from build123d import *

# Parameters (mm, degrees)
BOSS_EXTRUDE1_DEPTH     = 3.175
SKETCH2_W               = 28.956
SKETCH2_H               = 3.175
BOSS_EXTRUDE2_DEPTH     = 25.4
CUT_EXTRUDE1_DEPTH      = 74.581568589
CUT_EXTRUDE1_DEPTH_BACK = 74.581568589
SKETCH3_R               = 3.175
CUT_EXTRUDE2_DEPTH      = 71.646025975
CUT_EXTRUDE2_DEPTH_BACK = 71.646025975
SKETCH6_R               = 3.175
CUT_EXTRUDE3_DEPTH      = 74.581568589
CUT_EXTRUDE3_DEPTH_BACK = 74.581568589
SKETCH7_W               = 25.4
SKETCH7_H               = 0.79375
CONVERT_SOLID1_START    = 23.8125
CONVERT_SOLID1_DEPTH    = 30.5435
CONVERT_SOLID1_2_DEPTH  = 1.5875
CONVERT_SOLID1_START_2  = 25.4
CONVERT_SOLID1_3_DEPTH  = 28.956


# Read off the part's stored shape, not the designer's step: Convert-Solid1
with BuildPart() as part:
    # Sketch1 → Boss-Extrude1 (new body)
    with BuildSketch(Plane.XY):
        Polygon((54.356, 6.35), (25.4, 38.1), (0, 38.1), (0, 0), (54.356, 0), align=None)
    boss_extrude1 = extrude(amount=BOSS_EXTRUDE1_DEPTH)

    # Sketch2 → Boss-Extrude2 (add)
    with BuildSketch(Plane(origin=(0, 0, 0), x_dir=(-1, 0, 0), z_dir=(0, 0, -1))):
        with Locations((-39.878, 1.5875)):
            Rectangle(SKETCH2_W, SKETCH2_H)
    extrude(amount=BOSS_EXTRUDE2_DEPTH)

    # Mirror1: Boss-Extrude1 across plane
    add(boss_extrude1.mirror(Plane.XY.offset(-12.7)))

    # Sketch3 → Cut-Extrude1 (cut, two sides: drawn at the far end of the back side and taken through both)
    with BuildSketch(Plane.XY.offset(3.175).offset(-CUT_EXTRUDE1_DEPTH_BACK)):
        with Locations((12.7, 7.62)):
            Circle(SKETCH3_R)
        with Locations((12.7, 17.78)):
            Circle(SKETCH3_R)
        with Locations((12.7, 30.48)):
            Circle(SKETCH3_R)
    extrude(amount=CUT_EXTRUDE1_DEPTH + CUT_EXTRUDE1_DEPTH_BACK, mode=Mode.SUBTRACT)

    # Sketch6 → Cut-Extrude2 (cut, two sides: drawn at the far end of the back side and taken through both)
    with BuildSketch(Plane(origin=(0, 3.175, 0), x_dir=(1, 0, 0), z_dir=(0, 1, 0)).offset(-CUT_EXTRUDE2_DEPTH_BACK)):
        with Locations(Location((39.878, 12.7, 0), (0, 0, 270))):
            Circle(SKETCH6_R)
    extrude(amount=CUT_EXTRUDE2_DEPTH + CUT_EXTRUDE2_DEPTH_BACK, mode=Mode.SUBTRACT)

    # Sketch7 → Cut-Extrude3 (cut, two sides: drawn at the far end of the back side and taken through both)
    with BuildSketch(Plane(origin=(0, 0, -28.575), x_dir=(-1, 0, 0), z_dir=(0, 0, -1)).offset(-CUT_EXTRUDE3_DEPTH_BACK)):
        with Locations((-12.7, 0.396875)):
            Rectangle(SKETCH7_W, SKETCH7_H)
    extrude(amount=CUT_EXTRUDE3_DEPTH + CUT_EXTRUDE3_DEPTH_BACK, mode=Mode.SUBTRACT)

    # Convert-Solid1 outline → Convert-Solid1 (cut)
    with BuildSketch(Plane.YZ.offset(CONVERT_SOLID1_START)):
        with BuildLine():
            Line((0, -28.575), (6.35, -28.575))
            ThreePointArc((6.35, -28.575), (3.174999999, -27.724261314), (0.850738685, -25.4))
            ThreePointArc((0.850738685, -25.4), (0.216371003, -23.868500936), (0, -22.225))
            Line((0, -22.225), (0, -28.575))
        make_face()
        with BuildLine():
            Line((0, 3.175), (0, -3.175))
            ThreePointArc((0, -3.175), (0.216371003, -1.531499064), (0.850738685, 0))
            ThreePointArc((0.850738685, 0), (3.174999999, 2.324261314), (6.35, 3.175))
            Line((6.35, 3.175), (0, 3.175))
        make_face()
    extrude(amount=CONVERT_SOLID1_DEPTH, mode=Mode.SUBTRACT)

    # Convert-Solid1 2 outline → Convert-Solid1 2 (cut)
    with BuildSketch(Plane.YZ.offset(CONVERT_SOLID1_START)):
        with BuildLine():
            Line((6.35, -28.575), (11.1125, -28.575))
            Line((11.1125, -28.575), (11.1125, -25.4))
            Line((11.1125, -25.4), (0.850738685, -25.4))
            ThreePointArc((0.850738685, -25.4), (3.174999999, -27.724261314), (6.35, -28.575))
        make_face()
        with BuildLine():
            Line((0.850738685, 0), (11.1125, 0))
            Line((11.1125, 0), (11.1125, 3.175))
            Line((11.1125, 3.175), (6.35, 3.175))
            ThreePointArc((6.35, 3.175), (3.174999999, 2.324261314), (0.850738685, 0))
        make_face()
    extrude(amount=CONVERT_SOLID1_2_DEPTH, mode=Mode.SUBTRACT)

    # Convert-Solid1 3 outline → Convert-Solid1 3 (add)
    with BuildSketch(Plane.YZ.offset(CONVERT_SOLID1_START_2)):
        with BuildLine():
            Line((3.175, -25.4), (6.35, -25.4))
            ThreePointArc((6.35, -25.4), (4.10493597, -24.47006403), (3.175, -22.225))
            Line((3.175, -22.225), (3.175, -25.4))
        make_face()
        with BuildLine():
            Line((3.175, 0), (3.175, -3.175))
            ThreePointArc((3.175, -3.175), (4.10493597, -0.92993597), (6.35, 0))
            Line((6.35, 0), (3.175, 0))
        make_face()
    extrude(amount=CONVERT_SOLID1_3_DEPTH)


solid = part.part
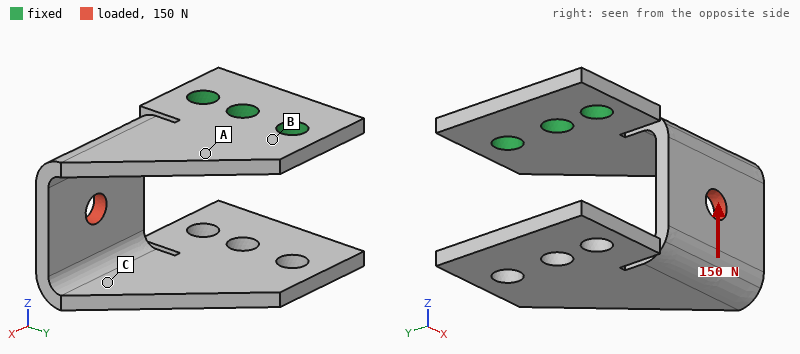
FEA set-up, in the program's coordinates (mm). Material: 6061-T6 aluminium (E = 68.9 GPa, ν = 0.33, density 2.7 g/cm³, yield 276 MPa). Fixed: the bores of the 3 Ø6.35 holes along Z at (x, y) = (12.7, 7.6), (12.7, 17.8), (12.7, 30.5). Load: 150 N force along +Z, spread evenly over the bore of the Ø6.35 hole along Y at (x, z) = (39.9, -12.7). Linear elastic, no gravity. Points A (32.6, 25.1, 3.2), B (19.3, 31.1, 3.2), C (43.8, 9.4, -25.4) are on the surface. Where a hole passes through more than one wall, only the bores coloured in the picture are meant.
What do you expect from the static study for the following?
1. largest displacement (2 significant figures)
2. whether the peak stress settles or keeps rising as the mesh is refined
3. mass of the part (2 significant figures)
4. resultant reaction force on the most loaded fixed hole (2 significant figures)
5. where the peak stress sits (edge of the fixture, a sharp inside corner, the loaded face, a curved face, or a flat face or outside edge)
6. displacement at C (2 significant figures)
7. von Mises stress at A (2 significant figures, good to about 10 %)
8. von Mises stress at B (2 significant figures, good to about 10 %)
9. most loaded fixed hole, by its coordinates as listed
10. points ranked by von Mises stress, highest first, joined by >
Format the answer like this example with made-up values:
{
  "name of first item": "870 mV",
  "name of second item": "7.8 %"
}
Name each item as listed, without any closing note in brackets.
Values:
{
  "largest displacement": "0.73 mm",
  "whether the peak stress settles or keeps rising as the mesh is refined": "keeps rising",
  "mass of the part": "30 g",
  "resultant reaction force on the most loaded fixed hole": "130 N",
  "where the peak stress sits": "a sharp inside corner",
  "displacement at C": "0.51 mm",
  "von Mises stress at A": "60 MPa",
  "von Mises stress at B": "32 MPa",
  "most loaded fixed hole, by its coordinates as listed": "(12.7, 7.6)",
  "points ranked by von Mises stress, highest first, joined by >": "A > B > C"
}
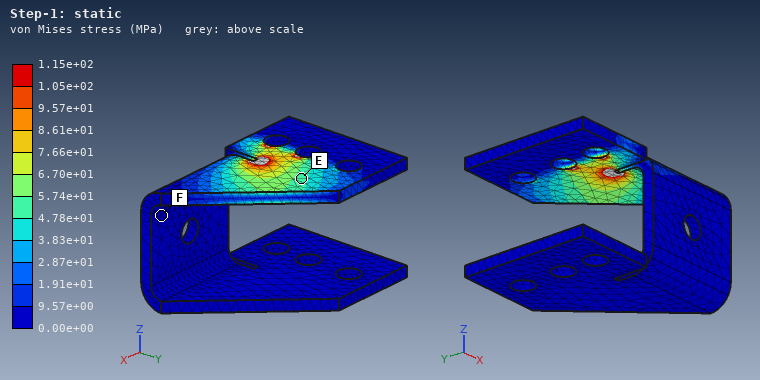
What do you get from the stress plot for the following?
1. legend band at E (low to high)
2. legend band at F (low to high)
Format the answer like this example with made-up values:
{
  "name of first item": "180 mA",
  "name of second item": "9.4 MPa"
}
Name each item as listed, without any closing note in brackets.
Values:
{
  "legend band at E": "4.78e+01 to 5.74e+01 MPa",
  "legend band at F": "0.00e+00 to 9.57e+00 MPa"
}
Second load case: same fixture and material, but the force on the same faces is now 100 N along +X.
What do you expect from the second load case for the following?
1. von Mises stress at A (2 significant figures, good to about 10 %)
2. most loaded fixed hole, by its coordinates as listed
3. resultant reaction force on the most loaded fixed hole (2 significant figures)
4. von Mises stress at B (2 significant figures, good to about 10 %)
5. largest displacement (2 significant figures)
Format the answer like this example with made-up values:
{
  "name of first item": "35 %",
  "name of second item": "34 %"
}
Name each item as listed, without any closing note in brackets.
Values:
{
  "von Mises stress at A": "33 MPa",
  "most loaded fixed hole, by its coordinates as listed": "(12.7, 17.8)",
  "resultant reaction force on the most loaded fixed hole": "110 N",
  "von Mises stress at B": "25 MPa",
  "largest displacement": "0.38 mm"
}
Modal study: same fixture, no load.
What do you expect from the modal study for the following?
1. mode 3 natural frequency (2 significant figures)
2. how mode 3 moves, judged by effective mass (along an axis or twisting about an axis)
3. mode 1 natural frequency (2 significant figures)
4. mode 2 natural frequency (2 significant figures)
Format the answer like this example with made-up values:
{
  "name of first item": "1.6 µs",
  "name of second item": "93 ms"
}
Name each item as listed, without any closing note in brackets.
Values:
{
  "mode 3 natural frequency": "960 Hz",
  "how mode 3 moves, judged by effective mass": "along Z",
  "mode 1 natural frequency": "440 Hz",
  "mode 2 natural frequency": "510 Hz"
}
